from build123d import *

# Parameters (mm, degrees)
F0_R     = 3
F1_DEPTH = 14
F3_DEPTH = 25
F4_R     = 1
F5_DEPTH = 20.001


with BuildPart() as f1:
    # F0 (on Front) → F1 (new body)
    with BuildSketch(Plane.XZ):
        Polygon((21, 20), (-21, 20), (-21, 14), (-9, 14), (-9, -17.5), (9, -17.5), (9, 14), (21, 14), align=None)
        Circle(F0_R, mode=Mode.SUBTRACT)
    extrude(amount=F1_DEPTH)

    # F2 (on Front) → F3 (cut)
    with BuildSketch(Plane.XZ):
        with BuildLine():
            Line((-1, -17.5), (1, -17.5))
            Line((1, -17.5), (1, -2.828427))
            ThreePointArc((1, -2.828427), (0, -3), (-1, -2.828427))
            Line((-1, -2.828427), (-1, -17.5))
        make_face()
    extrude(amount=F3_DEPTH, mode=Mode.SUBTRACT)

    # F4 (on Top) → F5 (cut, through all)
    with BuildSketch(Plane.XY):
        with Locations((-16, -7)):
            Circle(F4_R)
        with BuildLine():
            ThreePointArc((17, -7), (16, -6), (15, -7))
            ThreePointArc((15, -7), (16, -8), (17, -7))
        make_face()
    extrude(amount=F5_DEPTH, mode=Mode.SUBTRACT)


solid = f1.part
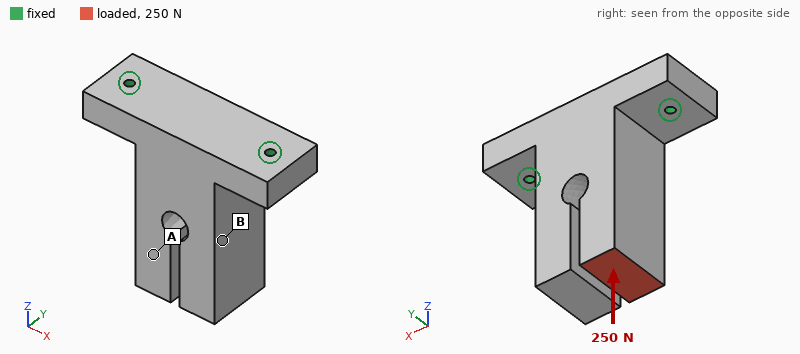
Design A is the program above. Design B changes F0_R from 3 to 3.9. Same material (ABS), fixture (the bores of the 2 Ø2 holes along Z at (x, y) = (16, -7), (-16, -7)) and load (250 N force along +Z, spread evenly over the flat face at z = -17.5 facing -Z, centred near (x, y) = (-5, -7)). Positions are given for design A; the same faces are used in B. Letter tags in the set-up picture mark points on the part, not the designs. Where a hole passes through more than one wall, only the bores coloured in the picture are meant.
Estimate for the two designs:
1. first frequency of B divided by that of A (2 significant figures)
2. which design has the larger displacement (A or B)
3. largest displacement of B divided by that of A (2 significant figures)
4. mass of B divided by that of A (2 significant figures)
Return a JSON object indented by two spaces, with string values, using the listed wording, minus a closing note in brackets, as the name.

{
  "first frequency of B divided by that of A": "1.0",
  "which design has the larger displacement": "B",
  "largest displacement of B divided by that of A": "1.3",
  "mass of B divided by that of A": "0.98"
}
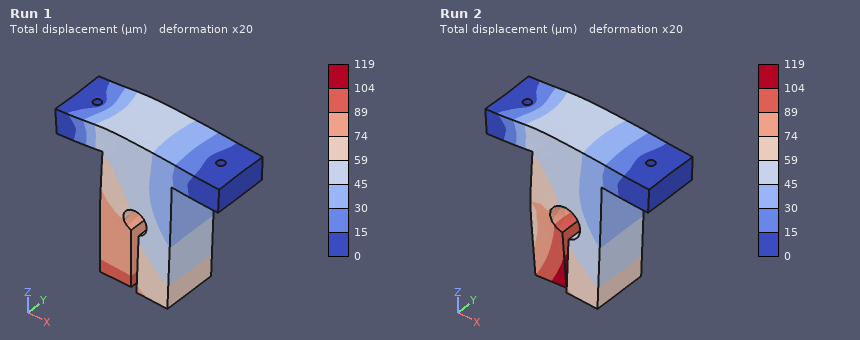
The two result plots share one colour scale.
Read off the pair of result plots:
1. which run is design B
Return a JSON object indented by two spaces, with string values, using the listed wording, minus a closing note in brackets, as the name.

{
  "which run is design B": "Run 2"
}
